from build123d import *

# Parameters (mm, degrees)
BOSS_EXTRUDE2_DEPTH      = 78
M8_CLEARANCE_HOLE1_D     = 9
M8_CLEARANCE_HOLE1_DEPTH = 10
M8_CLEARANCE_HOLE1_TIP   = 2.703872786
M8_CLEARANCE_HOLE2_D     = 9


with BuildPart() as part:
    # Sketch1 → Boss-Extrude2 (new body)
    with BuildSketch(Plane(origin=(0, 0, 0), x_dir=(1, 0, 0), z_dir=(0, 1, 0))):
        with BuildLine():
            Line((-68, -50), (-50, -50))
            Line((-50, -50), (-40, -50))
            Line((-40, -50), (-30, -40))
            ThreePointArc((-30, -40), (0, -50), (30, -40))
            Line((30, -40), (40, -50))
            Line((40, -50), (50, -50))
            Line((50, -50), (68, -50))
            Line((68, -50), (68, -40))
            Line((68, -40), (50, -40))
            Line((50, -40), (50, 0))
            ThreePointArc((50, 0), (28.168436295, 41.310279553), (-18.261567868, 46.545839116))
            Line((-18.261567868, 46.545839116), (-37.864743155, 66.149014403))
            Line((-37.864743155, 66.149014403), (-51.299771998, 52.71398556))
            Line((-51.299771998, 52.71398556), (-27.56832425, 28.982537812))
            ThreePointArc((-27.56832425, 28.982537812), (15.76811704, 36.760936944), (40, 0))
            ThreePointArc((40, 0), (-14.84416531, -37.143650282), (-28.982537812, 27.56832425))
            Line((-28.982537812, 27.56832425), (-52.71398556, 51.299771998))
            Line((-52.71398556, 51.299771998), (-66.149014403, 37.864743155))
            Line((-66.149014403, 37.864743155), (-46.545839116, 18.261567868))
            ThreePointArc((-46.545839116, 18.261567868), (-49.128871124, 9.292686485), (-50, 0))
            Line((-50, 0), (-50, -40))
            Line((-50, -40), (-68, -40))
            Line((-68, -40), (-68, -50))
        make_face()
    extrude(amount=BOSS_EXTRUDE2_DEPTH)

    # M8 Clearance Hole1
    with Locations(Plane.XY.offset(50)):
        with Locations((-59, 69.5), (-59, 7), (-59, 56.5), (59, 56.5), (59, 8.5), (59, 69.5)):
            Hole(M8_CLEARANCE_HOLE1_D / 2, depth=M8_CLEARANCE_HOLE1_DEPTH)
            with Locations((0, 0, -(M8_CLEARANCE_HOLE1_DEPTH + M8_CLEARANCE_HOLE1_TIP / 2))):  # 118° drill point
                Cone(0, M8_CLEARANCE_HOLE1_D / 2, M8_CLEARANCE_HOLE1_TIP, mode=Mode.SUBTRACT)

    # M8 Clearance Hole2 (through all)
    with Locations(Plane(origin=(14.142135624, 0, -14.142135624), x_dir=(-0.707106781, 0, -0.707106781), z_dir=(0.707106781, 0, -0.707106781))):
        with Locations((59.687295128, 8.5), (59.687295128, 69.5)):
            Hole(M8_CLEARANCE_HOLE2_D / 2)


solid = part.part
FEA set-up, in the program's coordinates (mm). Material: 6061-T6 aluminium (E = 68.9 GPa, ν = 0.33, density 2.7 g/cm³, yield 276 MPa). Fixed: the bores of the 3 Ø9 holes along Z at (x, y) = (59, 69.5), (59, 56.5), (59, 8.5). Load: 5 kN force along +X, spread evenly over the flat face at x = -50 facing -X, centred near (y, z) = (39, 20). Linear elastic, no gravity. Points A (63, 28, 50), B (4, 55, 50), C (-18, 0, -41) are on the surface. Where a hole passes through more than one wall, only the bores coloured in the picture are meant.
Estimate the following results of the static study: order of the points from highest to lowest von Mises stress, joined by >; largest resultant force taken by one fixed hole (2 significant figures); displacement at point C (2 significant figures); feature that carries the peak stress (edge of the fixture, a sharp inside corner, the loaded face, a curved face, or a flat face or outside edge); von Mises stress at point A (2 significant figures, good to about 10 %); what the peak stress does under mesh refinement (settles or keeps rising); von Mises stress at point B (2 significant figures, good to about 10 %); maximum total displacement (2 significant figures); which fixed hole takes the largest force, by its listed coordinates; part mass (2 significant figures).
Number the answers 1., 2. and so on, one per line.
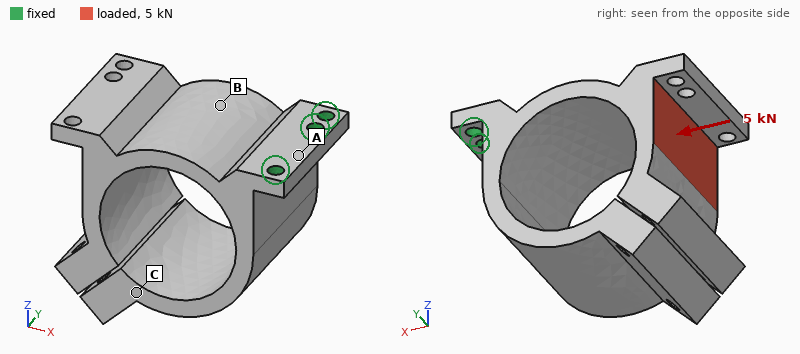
1. B > A > C
2. 2.1 kN
3. 0.41 mm
4. edge of the fixture
5. 20 MPa
6. keeps rising
7. 74 MPa
8. 2.1 mm
9. (59, 8.5)
10. 1.0 kg
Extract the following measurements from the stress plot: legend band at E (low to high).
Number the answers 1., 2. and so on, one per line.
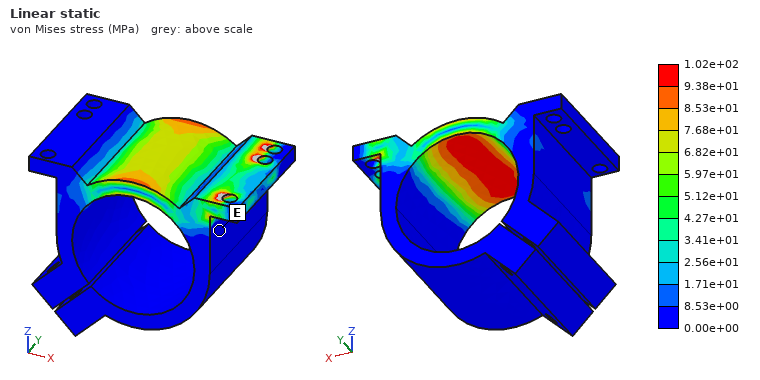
1. 0.00e+00 to 8.53e+00 MPa
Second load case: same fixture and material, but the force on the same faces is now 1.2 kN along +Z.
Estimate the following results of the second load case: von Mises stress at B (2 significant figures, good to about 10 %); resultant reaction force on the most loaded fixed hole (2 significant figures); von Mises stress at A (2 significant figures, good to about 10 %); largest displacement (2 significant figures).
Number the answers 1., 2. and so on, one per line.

1. 42 MPa
2. 590 N
3. 18 MPa
4. 1.4 mm
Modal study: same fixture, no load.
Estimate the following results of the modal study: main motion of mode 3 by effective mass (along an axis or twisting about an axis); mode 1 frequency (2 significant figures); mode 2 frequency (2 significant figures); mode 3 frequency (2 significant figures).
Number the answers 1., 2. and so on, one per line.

1. along Y
2. 240 Hz
3. 370 Hz
4. 580 Hz
